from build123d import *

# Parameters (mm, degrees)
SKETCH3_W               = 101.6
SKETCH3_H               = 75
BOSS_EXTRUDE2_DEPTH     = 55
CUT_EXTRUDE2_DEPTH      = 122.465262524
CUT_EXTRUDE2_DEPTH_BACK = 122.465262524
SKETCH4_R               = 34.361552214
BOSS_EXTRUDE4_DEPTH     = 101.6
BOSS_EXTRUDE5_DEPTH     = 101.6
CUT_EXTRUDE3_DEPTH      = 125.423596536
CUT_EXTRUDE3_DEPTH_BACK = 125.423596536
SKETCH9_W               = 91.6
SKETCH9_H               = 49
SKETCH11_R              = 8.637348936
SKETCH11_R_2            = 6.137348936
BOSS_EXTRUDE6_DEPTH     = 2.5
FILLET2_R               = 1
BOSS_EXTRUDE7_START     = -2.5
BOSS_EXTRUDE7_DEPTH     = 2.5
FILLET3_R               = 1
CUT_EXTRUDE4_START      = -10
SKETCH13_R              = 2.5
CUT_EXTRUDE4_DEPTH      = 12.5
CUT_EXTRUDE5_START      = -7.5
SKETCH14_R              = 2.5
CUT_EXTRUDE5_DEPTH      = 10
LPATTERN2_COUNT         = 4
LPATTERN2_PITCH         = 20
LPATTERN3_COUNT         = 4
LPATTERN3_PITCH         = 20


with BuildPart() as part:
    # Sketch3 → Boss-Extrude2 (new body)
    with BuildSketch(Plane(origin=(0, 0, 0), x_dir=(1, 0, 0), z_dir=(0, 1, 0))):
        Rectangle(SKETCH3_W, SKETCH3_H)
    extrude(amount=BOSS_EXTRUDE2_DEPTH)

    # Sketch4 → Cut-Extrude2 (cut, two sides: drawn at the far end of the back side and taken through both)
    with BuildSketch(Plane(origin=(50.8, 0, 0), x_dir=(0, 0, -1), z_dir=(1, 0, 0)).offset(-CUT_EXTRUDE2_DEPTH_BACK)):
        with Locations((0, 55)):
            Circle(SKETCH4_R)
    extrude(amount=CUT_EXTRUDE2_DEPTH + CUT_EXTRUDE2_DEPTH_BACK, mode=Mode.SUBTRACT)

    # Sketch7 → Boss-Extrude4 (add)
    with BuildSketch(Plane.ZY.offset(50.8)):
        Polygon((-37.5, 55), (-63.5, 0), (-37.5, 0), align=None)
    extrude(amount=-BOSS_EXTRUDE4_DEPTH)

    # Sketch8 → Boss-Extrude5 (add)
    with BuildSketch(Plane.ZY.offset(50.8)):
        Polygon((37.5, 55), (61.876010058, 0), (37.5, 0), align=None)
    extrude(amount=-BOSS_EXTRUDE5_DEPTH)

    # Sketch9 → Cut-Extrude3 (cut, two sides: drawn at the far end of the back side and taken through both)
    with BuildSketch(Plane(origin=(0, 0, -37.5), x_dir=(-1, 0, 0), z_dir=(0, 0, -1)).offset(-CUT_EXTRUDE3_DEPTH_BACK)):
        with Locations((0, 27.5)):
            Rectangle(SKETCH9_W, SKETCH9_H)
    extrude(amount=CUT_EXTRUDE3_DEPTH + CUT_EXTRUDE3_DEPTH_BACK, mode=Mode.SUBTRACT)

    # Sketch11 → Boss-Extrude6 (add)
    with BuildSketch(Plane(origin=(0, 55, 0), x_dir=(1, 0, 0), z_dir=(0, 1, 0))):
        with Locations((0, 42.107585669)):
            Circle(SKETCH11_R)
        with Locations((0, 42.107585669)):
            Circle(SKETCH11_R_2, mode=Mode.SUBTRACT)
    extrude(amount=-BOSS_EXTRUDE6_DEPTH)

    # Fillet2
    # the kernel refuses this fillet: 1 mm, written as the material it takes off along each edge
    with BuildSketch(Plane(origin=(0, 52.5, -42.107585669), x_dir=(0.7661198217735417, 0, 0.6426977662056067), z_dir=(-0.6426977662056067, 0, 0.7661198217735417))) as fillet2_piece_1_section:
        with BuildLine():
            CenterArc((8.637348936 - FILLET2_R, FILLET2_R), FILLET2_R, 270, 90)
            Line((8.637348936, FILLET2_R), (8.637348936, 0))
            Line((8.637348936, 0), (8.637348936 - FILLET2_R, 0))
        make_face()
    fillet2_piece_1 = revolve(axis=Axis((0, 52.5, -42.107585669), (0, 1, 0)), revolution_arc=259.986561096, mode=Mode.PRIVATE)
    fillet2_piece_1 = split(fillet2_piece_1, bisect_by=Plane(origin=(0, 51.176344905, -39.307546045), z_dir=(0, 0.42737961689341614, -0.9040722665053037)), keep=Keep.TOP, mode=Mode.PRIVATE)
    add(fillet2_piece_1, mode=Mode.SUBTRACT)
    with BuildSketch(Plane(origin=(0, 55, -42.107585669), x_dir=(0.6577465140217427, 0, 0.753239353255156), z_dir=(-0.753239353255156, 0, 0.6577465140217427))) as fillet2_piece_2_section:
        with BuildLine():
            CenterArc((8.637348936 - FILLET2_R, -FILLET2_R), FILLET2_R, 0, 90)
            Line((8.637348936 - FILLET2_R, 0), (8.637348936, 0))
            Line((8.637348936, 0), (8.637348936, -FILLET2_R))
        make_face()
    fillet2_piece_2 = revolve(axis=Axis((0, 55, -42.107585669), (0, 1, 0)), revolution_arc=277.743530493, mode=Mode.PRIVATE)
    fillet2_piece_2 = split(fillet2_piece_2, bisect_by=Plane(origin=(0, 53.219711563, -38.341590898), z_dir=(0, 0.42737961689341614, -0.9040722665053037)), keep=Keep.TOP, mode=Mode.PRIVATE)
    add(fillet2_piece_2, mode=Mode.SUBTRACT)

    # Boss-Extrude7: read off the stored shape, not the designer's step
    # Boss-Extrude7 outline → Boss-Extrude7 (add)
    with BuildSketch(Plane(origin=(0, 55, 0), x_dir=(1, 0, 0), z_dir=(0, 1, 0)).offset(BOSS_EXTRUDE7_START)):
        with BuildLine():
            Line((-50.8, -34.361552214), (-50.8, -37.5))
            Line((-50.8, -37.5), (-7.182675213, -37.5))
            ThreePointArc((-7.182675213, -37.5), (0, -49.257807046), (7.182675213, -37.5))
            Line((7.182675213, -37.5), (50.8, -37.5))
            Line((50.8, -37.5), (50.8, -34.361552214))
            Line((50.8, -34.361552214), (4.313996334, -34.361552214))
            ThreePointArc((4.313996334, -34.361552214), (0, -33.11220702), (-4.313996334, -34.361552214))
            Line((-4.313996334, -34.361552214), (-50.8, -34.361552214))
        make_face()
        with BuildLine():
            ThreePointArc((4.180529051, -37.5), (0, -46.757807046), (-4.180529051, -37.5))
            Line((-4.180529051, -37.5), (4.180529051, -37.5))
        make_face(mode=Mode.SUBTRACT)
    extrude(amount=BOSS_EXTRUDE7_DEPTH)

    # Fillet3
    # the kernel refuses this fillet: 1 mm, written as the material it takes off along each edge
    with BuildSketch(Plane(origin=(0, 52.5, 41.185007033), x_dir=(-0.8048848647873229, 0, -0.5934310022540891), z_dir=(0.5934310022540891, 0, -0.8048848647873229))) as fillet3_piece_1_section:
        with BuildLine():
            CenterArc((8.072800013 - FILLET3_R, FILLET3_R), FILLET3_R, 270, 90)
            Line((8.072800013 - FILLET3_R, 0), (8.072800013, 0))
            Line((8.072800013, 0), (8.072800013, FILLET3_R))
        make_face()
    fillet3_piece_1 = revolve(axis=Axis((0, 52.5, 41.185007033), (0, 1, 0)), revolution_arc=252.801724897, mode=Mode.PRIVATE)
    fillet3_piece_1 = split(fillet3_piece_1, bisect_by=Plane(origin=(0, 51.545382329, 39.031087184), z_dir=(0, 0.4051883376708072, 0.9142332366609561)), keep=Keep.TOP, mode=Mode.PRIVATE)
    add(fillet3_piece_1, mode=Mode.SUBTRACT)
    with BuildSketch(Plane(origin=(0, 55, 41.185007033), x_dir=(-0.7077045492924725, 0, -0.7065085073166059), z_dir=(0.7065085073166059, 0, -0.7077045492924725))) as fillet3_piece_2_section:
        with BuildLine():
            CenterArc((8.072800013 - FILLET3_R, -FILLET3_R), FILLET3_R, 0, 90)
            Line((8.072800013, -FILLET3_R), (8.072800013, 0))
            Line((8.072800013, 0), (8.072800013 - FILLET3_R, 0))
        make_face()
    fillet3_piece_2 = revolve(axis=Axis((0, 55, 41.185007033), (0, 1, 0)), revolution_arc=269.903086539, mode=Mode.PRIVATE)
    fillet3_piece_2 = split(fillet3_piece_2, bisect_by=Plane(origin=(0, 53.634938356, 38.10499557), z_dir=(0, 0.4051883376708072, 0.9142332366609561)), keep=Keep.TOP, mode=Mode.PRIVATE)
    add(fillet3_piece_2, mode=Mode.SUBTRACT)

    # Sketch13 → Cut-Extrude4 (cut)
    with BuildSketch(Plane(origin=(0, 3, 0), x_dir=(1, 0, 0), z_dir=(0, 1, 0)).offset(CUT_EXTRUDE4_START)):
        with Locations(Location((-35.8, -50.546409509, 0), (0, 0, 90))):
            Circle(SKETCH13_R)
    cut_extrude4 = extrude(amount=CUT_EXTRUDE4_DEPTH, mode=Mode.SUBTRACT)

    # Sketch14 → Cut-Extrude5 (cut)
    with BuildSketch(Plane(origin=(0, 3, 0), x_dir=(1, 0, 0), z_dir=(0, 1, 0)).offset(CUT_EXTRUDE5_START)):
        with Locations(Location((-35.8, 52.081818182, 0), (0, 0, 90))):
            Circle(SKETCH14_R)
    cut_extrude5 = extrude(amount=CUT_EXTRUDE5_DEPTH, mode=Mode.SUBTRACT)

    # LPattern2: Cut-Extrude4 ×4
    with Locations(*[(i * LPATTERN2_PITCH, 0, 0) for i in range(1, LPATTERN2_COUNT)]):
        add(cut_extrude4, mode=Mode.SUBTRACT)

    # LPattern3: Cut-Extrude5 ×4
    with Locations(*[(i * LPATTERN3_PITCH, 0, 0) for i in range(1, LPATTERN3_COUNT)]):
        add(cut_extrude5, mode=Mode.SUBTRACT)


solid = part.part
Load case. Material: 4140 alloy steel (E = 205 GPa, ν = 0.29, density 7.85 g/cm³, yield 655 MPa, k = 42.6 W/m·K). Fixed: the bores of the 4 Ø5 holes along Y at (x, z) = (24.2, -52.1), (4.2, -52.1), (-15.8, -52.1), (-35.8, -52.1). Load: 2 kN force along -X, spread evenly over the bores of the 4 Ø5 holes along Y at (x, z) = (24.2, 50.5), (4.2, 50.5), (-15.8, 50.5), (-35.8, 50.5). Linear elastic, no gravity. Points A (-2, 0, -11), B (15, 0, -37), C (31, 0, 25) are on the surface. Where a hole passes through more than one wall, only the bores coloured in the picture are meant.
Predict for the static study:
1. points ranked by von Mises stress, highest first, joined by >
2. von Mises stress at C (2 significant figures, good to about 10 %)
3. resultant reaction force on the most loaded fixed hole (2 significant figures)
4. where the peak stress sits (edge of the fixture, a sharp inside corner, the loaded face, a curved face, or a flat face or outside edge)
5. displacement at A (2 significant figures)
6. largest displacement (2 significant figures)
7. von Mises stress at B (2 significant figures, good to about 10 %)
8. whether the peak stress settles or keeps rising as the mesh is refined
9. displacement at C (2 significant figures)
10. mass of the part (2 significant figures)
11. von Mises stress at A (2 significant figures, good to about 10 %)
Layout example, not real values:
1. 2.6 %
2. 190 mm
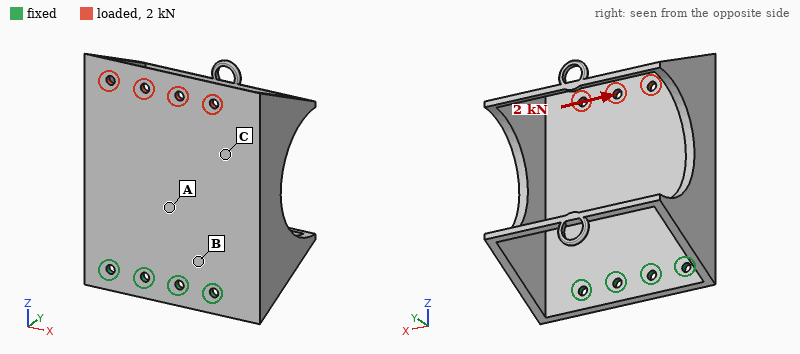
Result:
1. B > A > C
2. 9.8 MPa
3. 3.1 kN
4. edge of the fixture
5. 11 µm
6. 42 µm
7. 33 MPa
8. keeps rising
9. 26 µm
10. 570 g
11. 21 MPa
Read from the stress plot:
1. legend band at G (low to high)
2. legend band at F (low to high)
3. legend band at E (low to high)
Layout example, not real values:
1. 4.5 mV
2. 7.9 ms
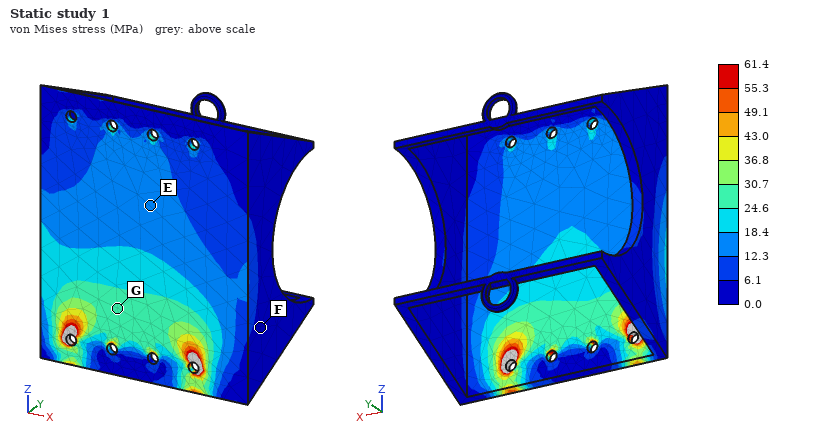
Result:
1. 24.6 to 30.7 MPa
2. 0.0 to 6.1 MPa
3. 12.3 to 18.4 MPa
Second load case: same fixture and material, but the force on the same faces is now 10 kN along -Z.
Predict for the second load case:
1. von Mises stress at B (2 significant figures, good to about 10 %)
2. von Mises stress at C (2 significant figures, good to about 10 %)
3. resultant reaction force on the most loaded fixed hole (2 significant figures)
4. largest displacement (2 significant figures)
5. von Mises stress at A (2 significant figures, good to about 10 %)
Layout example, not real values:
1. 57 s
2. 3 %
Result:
1. 37 MPa
2. 28 MPa
3. 3.0 kN
4. 39 µm
5. 42 MPa
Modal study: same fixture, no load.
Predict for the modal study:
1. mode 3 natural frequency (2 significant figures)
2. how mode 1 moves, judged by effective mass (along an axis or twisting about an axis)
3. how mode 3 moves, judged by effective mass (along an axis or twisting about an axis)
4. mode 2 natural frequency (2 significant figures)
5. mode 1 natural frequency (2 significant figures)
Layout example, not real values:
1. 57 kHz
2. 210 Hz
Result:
1. 1000 Hz
2. along Y
3. along X
4. 360 Hz
5. 230 Hz
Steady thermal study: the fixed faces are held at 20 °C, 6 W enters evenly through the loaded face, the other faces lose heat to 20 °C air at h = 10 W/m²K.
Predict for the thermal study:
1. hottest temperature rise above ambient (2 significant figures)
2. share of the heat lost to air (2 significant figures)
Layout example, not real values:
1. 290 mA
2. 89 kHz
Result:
1. 25 K
2. 61 %
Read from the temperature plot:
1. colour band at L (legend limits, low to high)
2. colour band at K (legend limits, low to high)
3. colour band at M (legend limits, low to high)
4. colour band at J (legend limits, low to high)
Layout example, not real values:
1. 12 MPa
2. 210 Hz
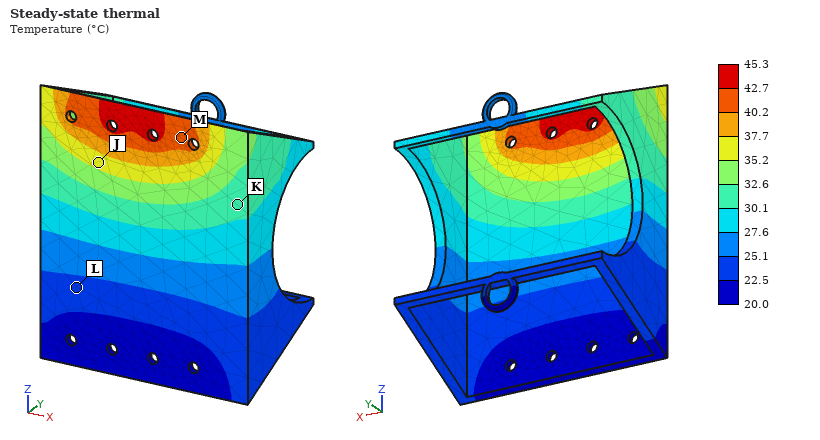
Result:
1. 22.5 to 25.1 °C
2. 30.1 to 32.6 °C
3. 40.2 to 42.7 °C
4. 35.2 to 37.7 °C
